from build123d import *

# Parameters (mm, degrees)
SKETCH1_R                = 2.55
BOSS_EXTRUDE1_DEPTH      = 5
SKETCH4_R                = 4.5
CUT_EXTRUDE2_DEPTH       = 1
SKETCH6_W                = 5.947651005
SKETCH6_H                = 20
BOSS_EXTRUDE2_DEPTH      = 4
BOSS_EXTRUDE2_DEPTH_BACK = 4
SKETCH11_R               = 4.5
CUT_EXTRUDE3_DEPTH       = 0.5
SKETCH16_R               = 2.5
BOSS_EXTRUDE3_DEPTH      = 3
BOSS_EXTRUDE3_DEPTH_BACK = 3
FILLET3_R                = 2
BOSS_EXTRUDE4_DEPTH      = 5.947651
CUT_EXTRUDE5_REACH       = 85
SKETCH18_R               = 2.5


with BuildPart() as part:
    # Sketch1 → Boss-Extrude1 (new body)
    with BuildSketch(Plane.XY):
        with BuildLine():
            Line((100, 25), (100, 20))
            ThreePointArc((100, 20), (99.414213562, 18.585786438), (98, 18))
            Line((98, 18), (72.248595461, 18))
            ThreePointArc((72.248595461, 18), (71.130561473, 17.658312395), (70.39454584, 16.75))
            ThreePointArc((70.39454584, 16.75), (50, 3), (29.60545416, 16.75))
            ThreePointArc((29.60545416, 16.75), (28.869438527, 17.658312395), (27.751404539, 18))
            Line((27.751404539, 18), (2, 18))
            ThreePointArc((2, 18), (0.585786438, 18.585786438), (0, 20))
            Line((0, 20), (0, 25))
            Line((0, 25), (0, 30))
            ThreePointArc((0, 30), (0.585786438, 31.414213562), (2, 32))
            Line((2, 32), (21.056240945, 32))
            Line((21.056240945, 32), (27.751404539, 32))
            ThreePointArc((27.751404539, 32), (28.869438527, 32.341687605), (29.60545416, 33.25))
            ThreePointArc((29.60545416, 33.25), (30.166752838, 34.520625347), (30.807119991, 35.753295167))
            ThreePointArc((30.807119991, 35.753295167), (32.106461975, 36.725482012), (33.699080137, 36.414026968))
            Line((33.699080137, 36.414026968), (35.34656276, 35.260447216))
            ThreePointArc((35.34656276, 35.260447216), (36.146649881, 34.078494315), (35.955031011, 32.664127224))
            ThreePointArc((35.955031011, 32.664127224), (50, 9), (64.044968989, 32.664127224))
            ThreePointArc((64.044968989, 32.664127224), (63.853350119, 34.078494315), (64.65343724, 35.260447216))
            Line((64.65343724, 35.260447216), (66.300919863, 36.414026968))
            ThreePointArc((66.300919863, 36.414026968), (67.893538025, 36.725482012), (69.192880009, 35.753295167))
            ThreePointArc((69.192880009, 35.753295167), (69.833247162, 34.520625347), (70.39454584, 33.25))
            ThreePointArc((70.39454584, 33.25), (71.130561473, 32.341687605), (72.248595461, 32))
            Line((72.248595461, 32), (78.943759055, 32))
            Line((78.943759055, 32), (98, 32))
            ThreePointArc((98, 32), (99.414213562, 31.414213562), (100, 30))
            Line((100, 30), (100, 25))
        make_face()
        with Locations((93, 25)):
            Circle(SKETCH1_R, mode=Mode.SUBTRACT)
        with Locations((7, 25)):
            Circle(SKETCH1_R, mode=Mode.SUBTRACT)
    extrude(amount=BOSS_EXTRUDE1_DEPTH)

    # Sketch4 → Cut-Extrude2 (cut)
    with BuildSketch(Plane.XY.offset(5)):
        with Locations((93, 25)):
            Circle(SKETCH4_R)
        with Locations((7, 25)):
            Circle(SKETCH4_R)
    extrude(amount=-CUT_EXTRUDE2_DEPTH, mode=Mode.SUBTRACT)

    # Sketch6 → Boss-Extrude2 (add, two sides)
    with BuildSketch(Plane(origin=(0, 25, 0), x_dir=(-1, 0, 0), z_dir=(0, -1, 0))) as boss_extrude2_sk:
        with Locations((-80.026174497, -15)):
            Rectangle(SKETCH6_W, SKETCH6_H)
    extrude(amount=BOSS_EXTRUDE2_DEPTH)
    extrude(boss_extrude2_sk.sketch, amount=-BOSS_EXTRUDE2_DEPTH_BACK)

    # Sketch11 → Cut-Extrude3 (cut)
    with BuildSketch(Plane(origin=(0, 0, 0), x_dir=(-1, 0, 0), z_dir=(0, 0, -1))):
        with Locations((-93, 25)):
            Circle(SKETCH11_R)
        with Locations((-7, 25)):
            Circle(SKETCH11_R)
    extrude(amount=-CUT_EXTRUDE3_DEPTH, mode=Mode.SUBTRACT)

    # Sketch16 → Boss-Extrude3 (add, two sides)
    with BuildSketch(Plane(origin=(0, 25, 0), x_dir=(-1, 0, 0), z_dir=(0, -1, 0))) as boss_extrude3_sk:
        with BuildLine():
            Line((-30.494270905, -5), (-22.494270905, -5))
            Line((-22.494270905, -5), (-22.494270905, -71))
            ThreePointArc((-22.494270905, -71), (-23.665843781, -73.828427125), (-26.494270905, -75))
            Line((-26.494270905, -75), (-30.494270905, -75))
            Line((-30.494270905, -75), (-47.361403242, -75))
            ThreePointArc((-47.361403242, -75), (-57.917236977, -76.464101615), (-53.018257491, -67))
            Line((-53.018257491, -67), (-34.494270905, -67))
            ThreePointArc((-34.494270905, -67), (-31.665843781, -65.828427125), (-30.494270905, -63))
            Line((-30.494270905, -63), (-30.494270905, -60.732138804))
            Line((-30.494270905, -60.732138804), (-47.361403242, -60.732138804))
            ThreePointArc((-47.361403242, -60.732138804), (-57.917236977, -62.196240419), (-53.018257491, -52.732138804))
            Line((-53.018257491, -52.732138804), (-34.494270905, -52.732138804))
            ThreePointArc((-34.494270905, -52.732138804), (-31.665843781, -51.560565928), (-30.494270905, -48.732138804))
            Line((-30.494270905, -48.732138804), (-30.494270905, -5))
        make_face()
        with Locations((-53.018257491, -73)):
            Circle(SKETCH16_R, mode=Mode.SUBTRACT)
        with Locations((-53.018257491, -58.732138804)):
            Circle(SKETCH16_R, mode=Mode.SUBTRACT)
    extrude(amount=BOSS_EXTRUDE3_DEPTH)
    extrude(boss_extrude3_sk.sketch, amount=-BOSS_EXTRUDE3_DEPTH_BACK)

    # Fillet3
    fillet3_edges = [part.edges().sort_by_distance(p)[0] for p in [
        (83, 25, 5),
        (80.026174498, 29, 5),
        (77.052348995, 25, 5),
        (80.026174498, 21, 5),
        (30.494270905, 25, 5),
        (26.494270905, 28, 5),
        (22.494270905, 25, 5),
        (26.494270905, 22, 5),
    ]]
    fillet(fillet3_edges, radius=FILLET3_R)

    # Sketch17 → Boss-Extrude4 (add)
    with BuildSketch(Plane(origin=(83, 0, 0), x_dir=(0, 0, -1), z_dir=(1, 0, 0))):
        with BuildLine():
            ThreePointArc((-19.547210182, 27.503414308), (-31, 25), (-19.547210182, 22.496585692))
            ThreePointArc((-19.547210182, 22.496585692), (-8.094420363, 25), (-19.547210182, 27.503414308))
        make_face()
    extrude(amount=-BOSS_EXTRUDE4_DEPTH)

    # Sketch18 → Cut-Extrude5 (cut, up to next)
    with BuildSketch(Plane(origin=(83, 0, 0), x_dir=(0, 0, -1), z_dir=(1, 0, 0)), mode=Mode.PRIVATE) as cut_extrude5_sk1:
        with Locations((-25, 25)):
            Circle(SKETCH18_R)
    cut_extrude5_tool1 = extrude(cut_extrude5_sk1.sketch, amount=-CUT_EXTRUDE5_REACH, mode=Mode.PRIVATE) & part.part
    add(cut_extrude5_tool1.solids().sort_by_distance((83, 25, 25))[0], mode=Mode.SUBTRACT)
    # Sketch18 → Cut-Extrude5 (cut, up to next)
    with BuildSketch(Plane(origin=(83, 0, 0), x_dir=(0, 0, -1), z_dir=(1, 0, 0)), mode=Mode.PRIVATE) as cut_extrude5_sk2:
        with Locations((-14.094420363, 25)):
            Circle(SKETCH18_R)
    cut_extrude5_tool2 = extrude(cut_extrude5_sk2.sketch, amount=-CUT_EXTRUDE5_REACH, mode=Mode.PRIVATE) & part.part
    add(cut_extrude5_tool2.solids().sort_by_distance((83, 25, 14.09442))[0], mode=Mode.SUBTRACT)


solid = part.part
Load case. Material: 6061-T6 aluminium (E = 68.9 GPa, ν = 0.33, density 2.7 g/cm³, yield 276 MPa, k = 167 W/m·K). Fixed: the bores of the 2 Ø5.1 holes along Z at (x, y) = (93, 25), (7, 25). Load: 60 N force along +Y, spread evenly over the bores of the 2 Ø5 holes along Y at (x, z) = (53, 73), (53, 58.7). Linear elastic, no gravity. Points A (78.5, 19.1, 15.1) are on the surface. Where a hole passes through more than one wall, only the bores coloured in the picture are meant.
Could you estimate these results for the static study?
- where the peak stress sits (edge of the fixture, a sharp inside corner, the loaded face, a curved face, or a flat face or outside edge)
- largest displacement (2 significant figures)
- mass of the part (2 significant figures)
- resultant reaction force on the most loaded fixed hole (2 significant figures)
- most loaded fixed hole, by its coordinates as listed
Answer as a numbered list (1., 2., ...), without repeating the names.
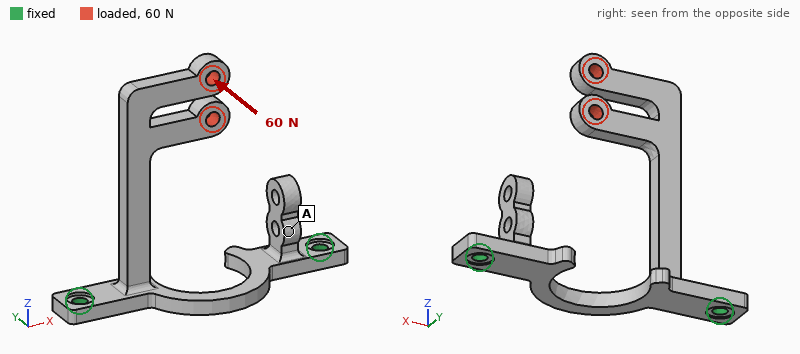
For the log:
1. a curved face
2. 1.3 mm
3. 37 g
4. 55 N
5. (7, 25)
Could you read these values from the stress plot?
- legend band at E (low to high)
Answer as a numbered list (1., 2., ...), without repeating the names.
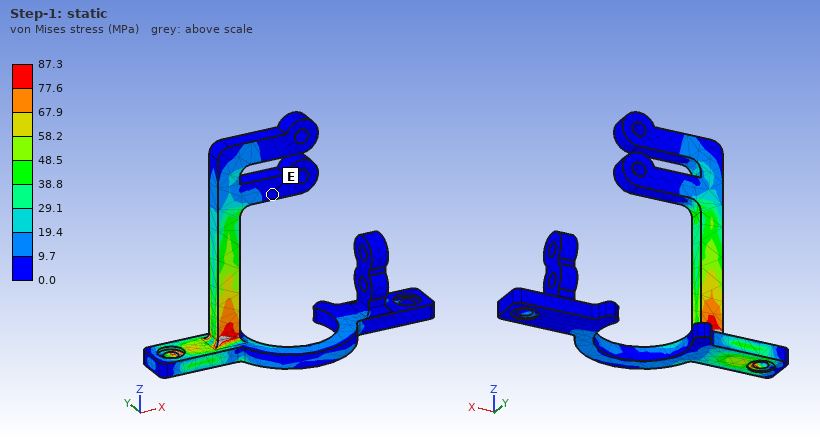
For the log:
1. 0.0 to 9.7 MPa
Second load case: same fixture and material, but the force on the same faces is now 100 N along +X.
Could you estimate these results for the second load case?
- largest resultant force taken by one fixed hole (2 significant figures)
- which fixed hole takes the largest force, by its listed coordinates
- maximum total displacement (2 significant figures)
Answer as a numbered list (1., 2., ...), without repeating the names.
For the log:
1. 110 N
2. (7, 25)
3. 1.3 mm
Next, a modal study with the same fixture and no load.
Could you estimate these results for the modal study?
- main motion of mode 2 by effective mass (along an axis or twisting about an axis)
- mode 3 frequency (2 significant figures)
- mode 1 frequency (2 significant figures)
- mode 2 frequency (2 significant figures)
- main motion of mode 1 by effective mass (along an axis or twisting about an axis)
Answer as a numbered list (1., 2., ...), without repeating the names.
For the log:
1. along X
2. 1700 Hz
3. 400 Hz
4. 470 Hz
5. along Y
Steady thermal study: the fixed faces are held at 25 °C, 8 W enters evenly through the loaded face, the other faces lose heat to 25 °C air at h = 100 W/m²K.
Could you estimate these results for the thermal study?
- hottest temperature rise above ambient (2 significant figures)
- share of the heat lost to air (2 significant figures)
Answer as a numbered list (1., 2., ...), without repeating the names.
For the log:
1. 27 K
2. 80 %
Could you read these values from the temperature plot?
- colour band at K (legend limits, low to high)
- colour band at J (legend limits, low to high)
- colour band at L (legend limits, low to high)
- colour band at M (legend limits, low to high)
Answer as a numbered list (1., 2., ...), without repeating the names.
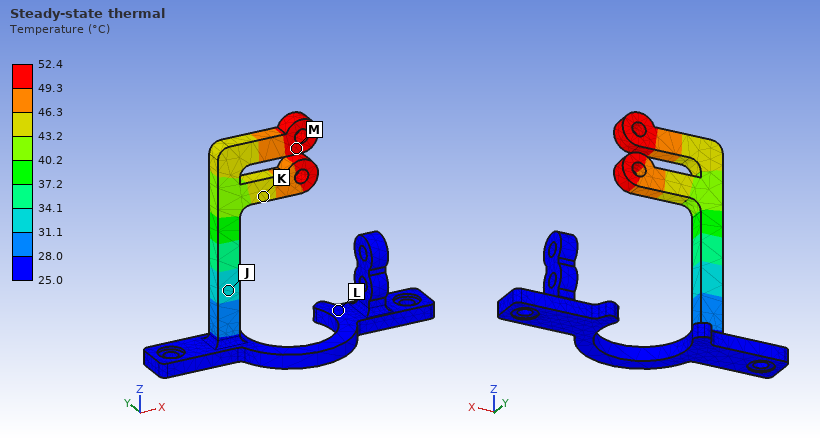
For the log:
1. 43.2 to 46.3 °C
2. 31.1 to 34.1 °C
3. 25.0 to 28.0 °C
4. 49.3 to 52.4 °C
